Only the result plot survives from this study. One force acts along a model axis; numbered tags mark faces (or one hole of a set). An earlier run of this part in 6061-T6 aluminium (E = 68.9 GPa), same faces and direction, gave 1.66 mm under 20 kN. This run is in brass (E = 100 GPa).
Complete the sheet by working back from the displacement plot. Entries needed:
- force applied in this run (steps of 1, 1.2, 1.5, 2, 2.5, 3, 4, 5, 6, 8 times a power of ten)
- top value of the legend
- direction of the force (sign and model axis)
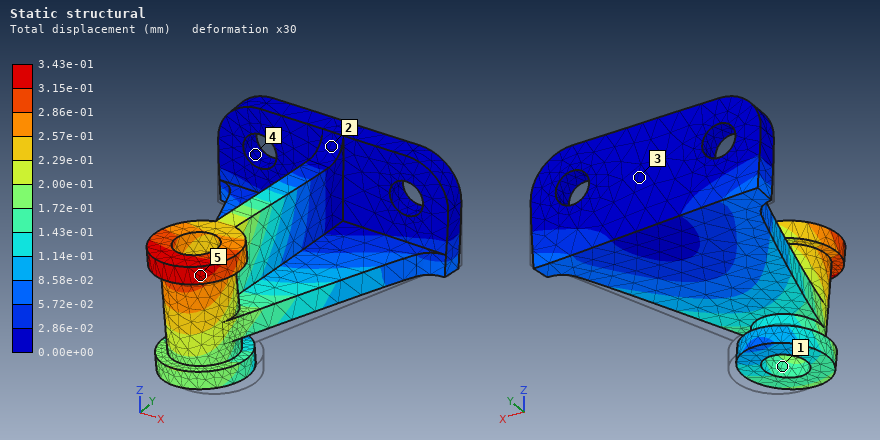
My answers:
6 kN
3.43e-01 mm
-X
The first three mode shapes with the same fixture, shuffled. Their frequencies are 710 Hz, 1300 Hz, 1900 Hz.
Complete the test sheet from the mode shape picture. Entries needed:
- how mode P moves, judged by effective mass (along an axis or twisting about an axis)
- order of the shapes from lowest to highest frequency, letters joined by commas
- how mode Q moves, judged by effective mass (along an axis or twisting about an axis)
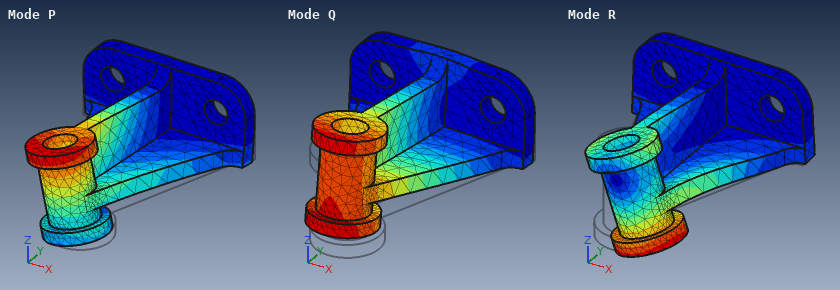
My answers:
along X
Q, P, R
along Z
